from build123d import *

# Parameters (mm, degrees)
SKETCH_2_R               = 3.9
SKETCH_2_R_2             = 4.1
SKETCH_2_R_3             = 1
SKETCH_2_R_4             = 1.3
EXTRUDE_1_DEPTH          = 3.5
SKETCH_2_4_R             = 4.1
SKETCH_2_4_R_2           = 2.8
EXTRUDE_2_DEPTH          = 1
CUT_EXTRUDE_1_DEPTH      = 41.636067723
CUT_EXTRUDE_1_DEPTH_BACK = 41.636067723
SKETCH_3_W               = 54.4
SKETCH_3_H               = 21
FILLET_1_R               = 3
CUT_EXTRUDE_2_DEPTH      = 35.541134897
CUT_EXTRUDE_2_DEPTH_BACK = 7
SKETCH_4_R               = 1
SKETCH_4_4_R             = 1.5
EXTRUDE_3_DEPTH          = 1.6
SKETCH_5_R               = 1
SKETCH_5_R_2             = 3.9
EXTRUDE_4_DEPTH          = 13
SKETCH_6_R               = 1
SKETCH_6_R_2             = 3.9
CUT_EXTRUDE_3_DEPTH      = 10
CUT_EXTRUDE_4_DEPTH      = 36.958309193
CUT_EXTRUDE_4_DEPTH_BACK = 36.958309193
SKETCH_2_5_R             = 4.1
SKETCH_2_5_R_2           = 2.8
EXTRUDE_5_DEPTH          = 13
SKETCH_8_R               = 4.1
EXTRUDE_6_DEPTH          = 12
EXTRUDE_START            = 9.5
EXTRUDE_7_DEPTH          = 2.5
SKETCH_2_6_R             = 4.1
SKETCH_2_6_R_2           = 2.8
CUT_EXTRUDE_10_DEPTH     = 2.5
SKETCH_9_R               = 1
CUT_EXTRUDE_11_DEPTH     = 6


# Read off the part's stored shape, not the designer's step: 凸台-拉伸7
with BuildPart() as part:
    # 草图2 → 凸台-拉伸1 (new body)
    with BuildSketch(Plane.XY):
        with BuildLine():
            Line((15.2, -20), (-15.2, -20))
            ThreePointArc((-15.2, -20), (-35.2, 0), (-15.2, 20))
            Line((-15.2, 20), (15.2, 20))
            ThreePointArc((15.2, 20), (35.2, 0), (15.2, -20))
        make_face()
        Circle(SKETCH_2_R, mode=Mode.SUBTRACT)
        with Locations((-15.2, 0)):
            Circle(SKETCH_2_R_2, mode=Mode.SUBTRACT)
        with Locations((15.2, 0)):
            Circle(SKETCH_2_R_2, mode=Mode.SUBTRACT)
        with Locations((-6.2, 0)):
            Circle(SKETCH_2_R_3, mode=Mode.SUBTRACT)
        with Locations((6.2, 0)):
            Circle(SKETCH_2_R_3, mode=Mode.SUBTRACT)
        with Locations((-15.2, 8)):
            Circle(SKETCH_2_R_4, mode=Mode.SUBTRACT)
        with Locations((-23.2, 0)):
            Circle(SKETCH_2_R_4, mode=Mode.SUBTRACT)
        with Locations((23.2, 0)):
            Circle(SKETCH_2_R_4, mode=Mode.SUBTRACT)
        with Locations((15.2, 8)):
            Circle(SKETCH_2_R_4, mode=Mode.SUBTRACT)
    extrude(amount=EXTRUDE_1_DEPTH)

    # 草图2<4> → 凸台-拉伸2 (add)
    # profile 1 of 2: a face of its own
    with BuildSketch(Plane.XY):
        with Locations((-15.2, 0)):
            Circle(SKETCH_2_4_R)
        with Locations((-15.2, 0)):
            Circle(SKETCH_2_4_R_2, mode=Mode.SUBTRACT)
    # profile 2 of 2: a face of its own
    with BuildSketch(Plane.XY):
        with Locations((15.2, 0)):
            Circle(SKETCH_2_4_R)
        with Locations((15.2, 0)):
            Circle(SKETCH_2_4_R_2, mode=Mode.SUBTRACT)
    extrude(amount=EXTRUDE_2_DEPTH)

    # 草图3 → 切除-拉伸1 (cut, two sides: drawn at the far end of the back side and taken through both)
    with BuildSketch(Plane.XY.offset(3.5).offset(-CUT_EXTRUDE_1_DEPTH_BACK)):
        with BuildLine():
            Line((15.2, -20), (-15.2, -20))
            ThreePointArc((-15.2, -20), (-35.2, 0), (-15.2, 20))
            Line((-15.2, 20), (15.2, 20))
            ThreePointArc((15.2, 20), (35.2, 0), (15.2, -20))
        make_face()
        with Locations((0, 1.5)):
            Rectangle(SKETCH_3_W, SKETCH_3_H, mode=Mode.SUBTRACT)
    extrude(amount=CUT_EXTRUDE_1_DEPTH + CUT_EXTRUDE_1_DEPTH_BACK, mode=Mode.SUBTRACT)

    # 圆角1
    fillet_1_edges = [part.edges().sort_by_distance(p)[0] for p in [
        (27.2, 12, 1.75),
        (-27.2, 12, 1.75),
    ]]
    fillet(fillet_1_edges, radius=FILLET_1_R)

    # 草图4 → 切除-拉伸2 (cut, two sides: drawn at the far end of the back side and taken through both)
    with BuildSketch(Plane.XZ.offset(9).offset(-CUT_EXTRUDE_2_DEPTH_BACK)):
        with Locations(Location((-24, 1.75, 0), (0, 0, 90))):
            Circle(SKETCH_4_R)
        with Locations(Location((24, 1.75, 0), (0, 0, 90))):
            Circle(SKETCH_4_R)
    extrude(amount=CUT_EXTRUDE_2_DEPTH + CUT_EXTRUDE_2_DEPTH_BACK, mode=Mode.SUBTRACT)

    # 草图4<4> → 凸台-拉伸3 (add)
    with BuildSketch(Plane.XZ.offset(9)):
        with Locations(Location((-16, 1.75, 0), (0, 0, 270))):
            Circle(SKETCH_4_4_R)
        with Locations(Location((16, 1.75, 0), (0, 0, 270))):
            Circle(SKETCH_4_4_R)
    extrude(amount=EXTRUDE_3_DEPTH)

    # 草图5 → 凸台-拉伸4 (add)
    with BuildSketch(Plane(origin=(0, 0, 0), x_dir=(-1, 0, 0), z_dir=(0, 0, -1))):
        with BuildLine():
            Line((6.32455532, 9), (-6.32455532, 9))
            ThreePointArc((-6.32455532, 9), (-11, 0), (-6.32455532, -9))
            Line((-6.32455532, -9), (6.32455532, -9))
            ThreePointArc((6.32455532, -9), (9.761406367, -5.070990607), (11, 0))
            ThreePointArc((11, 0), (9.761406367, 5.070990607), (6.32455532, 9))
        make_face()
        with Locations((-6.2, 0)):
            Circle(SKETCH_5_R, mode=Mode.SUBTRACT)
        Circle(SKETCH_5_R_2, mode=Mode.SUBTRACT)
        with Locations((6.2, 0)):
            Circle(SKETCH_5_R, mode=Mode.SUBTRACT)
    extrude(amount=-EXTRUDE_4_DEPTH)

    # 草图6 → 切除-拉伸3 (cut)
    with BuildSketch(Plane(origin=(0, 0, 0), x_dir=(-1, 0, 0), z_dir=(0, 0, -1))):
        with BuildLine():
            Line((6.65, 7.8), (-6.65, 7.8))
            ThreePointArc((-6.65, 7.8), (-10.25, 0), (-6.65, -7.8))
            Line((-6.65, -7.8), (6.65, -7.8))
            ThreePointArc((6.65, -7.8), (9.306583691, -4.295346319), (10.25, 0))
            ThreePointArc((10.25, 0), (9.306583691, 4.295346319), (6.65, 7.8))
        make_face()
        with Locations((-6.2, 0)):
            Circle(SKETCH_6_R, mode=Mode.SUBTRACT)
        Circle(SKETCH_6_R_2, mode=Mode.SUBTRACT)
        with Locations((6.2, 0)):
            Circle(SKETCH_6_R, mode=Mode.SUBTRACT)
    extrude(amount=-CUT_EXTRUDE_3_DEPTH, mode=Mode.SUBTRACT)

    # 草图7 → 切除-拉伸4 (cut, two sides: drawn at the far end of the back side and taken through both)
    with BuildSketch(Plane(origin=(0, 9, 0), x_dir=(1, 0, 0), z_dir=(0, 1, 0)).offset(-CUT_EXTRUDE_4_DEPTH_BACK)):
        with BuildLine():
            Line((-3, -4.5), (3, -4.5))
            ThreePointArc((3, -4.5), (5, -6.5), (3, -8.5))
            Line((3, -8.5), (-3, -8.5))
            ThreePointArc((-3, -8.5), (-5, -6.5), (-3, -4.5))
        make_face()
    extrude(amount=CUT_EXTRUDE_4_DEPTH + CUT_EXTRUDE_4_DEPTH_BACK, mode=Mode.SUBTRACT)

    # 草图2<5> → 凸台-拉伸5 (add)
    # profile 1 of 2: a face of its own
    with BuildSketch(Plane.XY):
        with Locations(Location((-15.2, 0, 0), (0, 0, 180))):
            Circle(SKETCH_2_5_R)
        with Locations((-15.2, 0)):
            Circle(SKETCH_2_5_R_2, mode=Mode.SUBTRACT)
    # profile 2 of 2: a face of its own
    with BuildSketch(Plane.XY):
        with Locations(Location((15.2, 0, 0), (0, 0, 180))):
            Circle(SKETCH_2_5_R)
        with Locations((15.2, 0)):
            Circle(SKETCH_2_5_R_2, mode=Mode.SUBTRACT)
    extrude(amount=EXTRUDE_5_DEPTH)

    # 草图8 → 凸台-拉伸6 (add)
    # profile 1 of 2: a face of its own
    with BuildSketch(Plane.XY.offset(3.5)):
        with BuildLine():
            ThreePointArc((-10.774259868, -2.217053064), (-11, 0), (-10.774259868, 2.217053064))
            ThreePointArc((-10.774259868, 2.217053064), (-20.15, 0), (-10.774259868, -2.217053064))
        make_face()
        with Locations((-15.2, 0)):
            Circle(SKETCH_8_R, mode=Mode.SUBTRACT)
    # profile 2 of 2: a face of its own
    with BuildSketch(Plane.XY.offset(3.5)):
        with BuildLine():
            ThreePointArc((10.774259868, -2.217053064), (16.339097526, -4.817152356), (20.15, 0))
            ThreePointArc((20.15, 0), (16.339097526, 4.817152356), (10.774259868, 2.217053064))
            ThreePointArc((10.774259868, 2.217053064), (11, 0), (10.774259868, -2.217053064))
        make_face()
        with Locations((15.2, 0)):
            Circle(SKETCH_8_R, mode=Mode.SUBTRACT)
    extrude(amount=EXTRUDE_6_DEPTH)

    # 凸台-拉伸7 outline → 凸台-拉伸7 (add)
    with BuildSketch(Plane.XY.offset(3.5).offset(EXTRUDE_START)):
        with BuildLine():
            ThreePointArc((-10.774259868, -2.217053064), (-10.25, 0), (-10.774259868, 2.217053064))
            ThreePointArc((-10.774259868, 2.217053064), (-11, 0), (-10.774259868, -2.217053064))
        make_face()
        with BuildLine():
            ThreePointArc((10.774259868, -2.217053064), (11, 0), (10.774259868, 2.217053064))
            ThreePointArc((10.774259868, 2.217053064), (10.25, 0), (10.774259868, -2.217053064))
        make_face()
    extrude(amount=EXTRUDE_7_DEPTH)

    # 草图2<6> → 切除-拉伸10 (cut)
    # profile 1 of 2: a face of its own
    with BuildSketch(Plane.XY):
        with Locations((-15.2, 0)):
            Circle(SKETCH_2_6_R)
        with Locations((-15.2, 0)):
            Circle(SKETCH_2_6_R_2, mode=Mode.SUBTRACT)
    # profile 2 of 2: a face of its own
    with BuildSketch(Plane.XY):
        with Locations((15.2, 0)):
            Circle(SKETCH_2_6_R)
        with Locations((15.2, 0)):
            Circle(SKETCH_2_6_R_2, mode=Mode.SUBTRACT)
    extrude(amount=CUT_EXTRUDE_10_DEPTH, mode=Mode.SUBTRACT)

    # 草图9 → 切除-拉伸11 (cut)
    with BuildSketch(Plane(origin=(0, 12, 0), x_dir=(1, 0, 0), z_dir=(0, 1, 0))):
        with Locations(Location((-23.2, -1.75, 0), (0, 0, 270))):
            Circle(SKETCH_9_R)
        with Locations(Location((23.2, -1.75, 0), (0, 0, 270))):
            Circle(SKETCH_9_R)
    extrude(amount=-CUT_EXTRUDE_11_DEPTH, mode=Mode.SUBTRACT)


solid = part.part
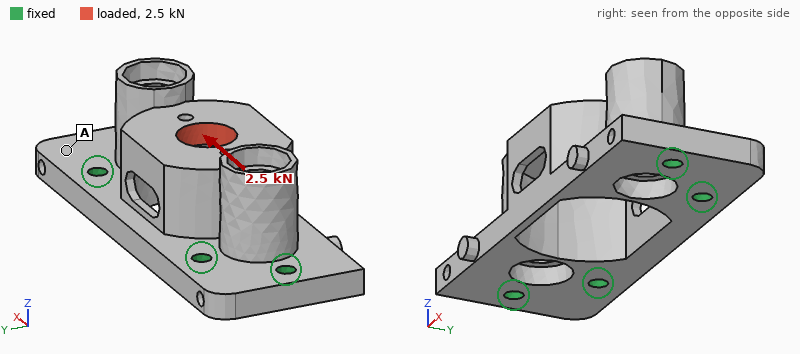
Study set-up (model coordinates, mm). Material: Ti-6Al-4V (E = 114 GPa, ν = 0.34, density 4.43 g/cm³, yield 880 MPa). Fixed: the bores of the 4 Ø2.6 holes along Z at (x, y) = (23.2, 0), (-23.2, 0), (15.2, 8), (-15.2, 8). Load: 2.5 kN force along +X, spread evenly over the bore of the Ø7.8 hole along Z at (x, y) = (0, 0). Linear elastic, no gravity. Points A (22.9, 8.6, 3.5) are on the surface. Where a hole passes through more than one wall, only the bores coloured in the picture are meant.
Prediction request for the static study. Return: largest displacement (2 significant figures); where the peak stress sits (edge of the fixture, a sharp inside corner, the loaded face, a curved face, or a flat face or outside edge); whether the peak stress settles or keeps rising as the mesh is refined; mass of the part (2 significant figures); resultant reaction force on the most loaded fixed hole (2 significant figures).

19 µm
a sharp inside corner
keeps rising
21 g
950 N
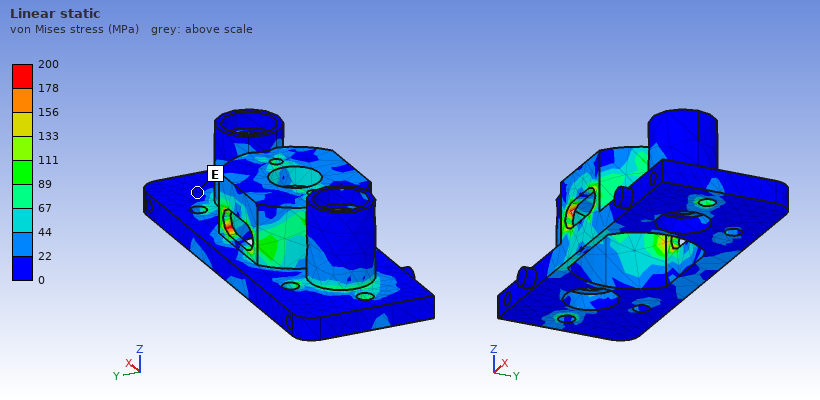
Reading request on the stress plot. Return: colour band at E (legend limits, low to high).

0 to 22 MPa
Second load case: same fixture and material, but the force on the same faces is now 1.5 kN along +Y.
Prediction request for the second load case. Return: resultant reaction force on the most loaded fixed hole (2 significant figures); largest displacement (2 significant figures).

950 N
55 µm
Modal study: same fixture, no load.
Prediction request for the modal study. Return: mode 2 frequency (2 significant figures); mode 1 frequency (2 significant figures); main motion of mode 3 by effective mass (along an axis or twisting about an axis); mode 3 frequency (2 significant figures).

20 kHz
9800 Hz
along Z
22 kHz
